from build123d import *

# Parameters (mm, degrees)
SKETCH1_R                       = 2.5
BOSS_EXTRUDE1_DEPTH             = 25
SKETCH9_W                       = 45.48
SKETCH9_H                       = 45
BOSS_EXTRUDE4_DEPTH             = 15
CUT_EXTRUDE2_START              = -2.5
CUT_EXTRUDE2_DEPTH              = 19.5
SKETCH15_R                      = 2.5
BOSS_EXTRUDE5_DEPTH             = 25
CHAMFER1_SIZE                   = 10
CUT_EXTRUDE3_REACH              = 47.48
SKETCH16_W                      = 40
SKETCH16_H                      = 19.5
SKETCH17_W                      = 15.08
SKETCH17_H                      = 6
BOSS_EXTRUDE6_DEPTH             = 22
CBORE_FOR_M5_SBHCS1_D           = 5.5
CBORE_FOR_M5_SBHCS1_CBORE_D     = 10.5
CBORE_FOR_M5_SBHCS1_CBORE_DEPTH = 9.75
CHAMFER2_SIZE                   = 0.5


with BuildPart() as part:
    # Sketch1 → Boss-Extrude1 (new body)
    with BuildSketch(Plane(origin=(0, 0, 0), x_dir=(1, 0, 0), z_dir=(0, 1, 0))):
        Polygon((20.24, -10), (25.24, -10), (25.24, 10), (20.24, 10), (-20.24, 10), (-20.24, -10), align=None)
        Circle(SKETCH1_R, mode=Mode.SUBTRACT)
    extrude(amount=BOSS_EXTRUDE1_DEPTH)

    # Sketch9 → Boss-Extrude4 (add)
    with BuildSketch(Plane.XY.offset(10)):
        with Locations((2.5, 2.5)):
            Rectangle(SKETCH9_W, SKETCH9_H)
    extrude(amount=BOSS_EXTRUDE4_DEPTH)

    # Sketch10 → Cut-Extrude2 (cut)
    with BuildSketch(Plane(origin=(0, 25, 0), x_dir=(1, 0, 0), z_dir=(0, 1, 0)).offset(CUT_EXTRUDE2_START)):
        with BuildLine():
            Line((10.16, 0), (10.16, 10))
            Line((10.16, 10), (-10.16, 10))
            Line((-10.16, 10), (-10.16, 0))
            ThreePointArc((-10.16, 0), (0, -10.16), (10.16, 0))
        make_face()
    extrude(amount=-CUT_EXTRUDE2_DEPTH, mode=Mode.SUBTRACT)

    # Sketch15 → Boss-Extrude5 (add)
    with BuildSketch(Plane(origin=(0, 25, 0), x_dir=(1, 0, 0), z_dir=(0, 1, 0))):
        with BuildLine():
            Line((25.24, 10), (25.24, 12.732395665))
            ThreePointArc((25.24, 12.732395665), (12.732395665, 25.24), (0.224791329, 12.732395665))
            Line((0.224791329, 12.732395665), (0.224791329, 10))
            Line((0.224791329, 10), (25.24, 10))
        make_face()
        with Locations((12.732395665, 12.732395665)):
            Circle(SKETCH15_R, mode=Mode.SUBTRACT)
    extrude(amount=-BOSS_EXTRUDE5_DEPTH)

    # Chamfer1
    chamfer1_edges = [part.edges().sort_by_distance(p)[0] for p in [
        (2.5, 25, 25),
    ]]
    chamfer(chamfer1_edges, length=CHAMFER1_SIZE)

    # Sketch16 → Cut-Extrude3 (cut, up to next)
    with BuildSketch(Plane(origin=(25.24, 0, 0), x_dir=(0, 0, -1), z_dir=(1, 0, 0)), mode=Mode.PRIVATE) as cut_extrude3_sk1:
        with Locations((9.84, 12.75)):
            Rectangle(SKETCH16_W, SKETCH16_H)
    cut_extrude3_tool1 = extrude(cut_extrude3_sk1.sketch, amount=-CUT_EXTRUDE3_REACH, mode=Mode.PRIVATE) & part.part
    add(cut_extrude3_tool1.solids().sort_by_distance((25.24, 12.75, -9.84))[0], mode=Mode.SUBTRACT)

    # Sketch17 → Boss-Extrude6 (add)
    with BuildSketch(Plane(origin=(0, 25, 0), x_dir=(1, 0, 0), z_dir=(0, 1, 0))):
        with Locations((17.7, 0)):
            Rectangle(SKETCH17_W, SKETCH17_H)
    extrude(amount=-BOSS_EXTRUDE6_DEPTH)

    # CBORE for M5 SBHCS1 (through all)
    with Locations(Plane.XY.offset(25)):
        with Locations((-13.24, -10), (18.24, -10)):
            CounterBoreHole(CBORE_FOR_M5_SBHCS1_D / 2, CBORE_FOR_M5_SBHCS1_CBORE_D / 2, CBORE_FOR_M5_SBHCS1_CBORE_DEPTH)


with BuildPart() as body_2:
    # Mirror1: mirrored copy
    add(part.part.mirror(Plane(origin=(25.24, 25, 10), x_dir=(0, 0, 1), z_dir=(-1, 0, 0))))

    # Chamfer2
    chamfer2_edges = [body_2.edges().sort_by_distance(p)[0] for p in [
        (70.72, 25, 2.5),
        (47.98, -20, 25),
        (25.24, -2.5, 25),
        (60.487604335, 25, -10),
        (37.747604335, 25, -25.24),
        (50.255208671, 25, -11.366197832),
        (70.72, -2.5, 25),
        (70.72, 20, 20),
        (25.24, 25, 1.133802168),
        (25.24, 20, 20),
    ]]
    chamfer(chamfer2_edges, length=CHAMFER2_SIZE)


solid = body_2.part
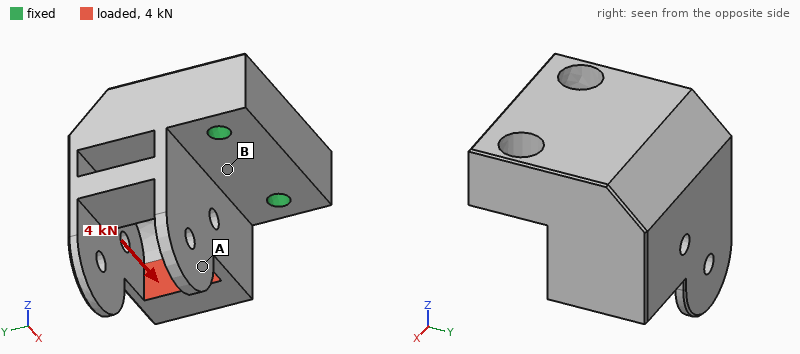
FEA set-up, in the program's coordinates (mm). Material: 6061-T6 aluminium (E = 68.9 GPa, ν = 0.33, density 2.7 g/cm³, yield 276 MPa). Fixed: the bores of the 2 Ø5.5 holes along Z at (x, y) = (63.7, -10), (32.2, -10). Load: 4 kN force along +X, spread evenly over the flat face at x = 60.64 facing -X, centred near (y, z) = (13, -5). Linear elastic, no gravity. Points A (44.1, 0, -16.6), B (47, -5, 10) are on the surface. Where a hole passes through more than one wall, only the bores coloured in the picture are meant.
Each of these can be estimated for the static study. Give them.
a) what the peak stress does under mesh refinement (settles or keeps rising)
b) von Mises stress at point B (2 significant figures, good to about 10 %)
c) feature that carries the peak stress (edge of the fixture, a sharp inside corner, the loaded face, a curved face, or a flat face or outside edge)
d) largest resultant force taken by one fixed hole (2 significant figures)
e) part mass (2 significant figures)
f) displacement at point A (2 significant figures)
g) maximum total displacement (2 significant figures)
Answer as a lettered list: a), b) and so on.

a) keeps rising
b) 47 MPa
c) edge of the fixture
d) 3.9 kN
e) 110 g
f) 0.050 mm
g) 0.10 mm
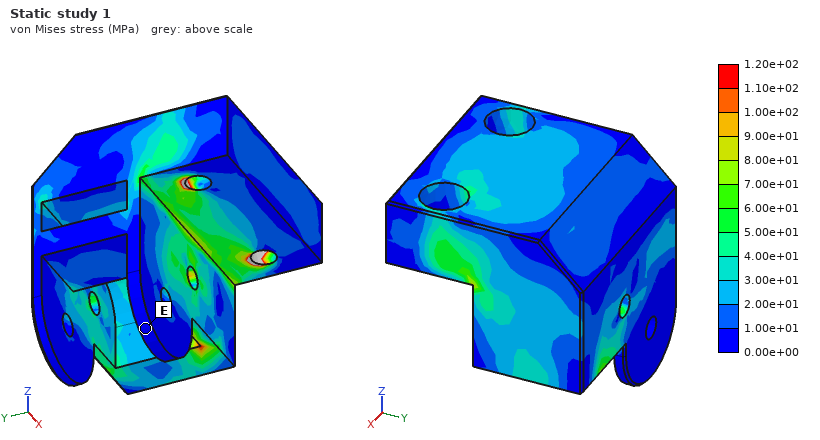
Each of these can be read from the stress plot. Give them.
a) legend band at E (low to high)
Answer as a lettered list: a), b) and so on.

a) 0.00e+00 to 1.00e+01 MPa
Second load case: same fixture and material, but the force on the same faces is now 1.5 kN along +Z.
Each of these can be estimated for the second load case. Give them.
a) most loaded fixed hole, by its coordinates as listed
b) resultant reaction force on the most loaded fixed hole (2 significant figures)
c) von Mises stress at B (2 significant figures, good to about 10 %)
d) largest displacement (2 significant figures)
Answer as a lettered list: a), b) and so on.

a) (63.7, -10)
b) 1.3 kN
c) 14 MPa
d) 0.11 mm
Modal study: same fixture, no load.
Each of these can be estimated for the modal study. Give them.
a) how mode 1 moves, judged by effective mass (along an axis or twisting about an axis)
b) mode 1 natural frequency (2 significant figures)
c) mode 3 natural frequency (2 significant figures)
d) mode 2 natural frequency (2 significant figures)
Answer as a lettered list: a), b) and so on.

a) along Z
b) 2600 Hz
c) 5000 Hz
d) 4500 Hz
